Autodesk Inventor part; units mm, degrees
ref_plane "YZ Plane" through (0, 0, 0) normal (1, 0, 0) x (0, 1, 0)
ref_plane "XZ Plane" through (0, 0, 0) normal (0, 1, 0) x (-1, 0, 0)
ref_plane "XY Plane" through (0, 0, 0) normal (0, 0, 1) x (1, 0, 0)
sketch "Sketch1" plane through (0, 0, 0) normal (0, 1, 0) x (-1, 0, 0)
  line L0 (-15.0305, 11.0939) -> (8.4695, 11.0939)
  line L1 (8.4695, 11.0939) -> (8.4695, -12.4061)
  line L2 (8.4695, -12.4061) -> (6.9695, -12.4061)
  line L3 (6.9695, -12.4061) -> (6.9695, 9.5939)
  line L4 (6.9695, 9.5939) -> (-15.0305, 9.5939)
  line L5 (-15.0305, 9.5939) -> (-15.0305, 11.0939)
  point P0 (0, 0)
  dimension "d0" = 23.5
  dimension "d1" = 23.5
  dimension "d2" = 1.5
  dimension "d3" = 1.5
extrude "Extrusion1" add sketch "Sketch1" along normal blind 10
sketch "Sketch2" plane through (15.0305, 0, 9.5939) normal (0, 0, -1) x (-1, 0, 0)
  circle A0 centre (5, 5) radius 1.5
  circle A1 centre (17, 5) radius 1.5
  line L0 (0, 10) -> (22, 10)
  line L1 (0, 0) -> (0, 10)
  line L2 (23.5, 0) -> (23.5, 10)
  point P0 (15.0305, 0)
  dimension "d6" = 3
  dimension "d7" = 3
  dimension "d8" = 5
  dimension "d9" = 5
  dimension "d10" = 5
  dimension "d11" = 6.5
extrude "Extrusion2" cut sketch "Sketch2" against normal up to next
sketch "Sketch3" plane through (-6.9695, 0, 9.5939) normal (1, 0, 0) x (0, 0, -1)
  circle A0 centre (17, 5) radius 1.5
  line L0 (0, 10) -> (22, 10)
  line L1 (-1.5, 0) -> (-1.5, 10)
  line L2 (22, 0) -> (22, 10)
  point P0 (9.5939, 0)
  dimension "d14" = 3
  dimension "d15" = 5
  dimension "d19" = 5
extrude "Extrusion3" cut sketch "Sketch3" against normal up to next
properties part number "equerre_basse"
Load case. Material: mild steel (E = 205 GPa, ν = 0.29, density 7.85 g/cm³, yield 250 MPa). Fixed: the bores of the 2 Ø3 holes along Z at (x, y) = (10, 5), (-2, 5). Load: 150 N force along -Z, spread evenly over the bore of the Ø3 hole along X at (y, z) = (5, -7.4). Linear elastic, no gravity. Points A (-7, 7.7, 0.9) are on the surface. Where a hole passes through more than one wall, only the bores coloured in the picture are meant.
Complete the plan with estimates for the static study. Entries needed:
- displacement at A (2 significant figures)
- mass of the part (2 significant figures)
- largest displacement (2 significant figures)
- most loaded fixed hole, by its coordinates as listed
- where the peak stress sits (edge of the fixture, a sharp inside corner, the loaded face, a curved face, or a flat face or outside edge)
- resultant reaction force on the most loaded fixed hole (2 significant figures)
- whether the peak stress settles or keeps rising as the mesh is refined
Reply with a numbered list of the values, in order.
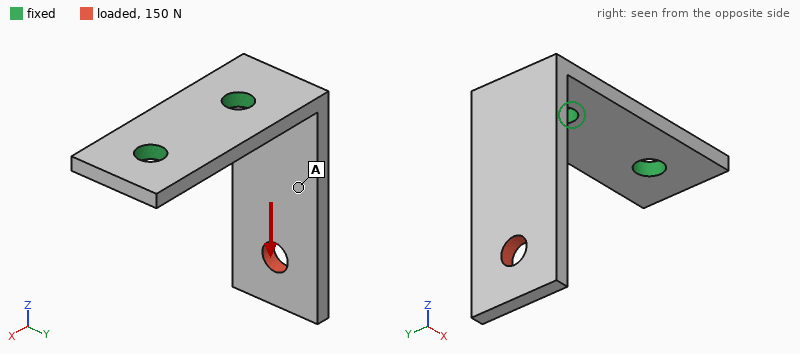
1. 32 µm
2. 5.1 g
3. 75 µm
4. (-2, 5)
5. edge of the fixture
6. 150 N
7. keeps rising
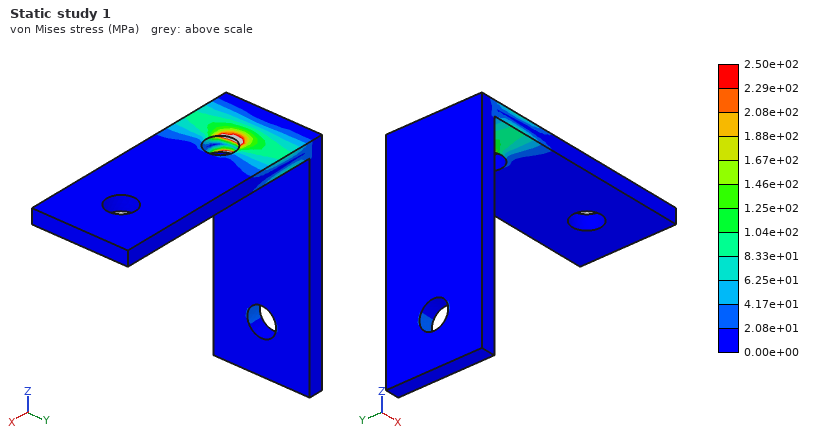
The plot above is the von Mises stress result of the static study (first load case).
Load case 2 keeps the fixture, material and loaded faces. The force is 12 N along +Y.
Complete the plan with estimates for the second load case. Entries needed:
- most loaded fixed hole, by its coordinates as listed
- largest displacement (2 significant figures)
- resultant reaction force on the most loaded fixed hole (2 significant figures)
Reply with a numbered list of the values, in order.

1. (-2, 5)
2. 22 µm
3. 15 N
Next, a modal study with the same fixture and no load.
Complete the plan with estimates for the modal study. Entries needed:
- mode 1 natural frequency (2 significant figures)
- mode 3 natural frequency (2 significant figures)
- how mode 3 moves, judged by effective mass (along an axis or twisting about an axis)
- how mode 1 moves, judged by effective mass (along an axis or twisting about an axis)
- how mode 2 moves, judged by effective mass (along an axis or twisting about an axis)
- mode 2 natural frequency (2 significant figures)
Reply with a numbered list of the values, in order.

1. 1900 Hz
2. 11 kHz
3. along Z
4. along X
5. along Y
6. 3600 Hz
